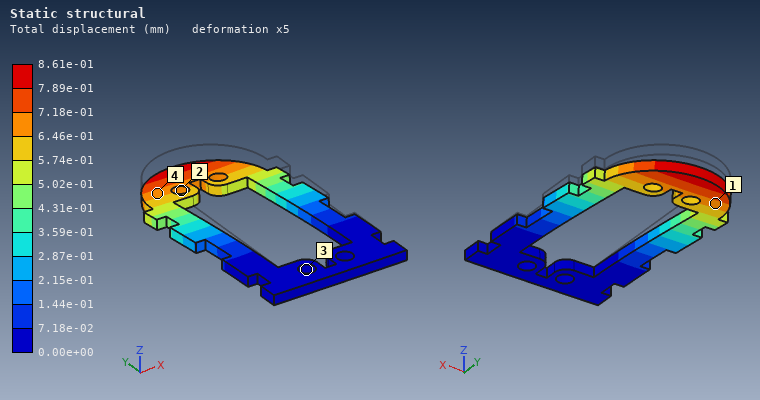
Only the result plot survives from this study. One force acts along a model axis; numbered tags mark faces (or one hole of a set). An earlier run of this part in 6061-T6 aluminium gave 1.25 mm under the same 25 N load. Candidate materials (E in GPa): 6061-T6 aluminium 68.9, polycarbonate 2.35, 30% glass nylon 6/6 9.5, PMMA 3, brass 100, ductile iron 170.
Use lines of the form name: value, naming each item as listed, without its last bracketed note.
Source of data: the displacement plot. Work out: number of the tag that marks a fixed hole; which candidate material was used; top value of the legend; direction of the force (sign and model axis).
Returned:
number of the tag that marks a fixed hole: 3
which candidate material was used: brass
top value of the legend: 8.61e-01 mm
direction of the force: -Z
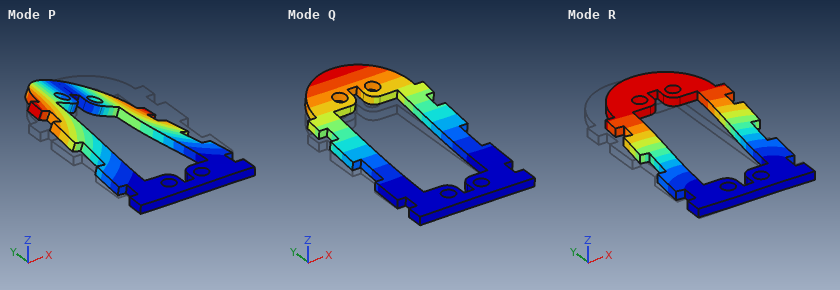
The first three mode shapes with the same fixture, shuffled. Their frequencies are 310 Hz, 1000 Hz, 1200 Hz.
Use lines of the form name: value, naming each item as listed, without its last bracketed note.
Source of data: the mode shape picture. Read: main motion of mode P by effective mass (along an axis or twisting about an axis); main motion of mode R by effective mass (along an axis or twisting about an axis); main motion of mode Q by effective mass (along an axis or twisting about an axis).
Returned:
main motion of mode P by effective mass: twisting about Y
main motion of mode R by effective mass: along X
main motion of mode Q by effective mass: along Z
